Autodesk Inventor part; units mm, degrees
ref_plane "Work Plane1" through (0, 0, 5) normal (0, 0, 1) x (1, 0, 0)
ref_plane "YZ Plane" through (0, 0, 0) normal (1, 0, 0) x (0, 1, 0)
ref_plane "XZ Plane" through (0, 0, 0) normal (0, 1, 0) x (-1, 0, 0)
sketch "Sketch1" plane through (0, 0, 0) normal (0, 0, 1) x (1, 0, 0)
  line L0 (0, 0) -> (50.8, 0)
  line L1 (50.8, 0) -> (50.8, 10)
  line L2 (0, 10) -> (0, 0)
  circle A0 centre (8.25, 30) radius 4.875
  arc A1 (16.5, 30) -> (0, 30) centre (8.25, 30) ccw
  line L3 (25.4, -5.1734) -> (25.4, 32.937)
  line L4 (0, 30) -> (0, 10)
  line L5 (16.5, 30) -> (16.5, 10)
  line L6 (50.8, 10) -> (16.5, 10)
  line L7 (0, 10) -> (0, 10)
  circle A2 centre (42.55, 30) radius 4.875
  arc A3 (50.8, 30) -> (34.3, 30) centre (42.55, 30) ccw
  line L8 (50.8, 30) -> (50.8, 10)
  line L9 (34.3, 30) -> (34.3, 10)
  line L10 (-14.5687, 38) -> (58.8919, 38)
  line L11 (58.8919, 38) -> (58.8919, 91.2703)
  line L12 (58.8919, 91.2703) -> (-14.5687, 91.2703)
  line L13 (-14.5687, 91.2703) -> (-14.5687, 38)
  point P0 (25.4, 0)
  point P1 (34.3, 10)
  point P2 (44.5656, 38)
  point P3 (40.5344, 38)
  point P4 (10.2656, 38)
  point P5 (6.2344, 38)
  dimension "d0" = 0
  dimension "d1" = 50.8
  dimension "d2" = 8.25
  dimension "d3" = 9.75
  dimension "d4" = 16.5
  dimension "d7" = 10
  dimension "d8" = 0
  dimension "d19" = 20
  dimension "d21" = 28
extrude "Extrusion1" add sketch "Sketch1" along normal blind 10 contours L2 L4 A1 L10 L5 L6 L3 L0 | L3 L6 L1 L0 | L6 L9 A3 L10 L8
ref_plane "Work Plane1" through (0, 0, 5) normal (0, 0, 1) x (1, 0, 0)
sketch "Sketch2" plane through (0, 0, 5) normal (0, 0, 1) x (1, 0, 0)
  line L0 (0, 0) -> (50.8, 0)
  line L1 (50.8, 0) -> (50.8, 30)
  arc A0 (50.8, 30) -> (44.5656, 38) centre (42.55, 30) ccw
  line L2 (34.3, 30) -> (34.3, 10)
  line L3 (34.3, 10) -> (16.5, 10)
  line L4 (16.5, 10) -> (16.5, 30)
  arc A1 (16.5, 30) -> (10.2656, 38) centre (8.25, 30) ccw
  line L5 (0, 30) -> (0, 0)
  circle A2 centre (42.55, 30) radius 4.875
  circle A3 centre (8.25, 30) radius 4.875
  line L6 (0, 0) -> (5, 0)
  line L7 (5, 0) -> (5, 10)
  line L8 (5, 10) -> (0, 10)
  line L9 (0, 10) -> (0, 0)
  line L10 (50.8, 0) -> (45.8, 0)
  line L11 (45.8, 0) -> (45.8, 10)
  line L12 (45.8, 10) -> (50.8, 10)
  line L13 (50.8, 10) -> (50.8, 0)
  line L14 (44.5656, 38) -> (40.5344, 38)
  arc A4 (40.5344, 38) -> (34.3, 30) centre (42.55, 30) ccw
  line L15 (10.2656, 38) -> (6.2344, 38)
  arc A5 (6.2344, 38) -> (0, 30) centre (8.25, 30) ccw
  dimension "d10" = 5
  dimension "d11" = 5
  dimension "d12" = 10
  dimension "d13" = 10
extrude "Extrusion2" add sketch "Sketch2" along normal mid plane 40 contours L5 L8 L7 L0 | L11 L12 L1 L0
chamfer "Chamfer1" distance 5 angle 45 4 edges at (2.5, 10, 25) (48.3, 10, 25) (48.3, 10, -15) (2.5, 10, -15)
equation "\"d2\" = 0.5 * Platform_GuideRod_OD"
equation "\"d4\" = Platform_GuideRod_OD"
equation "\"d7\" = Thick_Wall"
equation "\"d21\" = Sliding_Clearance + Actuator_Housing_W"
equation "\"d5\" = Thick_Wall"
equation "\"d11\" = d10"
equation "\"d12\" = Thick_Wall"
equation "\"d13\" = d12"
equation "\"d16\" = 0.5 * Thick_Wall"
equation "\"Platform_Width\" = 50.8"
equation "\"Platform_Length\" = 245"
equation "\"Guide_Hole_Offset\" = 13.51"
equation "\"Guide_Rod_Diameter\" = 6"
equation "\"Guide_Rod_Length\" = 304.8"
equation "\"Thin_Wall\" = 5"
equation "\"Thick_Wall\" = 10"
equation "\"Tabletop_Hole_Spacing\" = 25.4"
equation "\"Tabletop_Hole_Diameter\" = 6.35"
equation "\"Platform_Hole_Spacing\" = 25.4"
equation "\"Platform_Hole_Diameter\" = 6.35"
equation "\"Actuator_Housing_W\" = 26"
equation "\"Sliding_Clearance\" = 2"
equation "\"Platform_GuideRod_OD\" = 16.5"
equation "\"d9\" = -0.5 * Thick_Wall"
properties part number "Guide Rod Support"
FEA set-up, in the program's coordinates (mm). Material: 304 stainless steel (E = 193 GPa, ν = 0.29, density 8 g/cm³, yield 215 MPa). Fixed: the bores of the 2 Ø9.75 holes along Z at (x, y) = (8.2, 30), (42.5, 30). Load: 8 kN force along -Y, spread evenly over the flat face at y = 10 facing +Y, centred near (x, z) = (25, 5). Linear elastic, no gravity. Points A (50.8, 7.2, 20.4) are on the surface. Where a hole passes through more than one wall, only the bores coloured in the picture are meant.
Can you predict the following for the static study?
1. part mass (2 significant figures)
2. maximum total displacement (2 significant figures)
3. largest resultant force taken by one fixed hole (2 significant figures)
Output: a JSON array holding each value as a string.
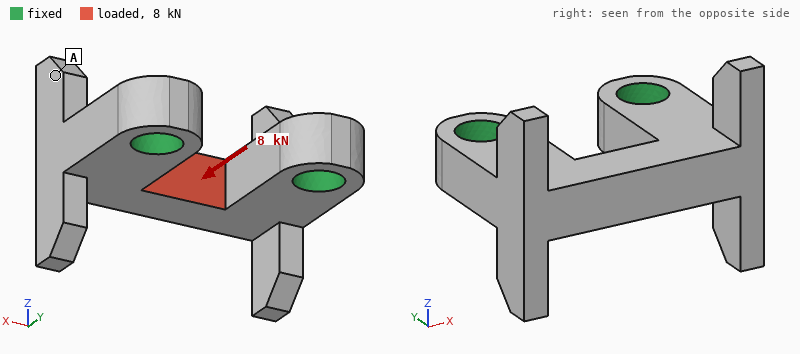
["120 g", "13 µm", "4.3 kN"]
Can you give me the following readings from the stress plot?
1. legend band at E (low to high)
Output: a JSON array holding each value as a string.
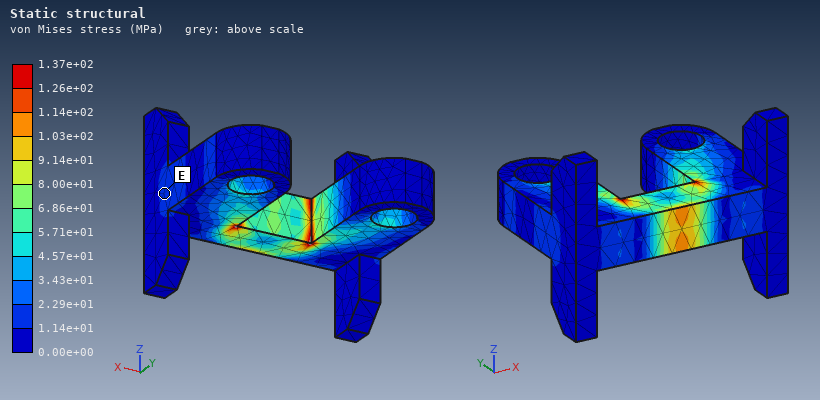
["1.14e+01 to 2.29e+01 MPa"]
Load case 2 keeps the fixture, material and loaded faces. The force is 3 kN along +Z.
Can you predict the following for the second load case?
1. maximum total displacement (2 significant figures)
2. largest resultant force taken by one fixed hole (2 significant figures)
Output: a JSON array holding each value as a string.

["25 µm", "1.5 kN"]
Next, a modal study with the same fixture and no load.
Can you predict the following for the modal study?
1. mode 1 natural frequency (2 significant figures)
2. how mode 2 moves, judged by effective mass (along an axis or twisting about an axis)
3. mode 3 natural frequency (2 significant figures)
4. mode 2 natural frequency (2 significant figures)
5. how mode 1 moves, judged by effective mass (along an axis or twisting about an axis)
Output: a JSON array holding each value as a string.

["6300 Hz", "twisting about Y", "10 kHz", "7700 Hz", "along Z"]
